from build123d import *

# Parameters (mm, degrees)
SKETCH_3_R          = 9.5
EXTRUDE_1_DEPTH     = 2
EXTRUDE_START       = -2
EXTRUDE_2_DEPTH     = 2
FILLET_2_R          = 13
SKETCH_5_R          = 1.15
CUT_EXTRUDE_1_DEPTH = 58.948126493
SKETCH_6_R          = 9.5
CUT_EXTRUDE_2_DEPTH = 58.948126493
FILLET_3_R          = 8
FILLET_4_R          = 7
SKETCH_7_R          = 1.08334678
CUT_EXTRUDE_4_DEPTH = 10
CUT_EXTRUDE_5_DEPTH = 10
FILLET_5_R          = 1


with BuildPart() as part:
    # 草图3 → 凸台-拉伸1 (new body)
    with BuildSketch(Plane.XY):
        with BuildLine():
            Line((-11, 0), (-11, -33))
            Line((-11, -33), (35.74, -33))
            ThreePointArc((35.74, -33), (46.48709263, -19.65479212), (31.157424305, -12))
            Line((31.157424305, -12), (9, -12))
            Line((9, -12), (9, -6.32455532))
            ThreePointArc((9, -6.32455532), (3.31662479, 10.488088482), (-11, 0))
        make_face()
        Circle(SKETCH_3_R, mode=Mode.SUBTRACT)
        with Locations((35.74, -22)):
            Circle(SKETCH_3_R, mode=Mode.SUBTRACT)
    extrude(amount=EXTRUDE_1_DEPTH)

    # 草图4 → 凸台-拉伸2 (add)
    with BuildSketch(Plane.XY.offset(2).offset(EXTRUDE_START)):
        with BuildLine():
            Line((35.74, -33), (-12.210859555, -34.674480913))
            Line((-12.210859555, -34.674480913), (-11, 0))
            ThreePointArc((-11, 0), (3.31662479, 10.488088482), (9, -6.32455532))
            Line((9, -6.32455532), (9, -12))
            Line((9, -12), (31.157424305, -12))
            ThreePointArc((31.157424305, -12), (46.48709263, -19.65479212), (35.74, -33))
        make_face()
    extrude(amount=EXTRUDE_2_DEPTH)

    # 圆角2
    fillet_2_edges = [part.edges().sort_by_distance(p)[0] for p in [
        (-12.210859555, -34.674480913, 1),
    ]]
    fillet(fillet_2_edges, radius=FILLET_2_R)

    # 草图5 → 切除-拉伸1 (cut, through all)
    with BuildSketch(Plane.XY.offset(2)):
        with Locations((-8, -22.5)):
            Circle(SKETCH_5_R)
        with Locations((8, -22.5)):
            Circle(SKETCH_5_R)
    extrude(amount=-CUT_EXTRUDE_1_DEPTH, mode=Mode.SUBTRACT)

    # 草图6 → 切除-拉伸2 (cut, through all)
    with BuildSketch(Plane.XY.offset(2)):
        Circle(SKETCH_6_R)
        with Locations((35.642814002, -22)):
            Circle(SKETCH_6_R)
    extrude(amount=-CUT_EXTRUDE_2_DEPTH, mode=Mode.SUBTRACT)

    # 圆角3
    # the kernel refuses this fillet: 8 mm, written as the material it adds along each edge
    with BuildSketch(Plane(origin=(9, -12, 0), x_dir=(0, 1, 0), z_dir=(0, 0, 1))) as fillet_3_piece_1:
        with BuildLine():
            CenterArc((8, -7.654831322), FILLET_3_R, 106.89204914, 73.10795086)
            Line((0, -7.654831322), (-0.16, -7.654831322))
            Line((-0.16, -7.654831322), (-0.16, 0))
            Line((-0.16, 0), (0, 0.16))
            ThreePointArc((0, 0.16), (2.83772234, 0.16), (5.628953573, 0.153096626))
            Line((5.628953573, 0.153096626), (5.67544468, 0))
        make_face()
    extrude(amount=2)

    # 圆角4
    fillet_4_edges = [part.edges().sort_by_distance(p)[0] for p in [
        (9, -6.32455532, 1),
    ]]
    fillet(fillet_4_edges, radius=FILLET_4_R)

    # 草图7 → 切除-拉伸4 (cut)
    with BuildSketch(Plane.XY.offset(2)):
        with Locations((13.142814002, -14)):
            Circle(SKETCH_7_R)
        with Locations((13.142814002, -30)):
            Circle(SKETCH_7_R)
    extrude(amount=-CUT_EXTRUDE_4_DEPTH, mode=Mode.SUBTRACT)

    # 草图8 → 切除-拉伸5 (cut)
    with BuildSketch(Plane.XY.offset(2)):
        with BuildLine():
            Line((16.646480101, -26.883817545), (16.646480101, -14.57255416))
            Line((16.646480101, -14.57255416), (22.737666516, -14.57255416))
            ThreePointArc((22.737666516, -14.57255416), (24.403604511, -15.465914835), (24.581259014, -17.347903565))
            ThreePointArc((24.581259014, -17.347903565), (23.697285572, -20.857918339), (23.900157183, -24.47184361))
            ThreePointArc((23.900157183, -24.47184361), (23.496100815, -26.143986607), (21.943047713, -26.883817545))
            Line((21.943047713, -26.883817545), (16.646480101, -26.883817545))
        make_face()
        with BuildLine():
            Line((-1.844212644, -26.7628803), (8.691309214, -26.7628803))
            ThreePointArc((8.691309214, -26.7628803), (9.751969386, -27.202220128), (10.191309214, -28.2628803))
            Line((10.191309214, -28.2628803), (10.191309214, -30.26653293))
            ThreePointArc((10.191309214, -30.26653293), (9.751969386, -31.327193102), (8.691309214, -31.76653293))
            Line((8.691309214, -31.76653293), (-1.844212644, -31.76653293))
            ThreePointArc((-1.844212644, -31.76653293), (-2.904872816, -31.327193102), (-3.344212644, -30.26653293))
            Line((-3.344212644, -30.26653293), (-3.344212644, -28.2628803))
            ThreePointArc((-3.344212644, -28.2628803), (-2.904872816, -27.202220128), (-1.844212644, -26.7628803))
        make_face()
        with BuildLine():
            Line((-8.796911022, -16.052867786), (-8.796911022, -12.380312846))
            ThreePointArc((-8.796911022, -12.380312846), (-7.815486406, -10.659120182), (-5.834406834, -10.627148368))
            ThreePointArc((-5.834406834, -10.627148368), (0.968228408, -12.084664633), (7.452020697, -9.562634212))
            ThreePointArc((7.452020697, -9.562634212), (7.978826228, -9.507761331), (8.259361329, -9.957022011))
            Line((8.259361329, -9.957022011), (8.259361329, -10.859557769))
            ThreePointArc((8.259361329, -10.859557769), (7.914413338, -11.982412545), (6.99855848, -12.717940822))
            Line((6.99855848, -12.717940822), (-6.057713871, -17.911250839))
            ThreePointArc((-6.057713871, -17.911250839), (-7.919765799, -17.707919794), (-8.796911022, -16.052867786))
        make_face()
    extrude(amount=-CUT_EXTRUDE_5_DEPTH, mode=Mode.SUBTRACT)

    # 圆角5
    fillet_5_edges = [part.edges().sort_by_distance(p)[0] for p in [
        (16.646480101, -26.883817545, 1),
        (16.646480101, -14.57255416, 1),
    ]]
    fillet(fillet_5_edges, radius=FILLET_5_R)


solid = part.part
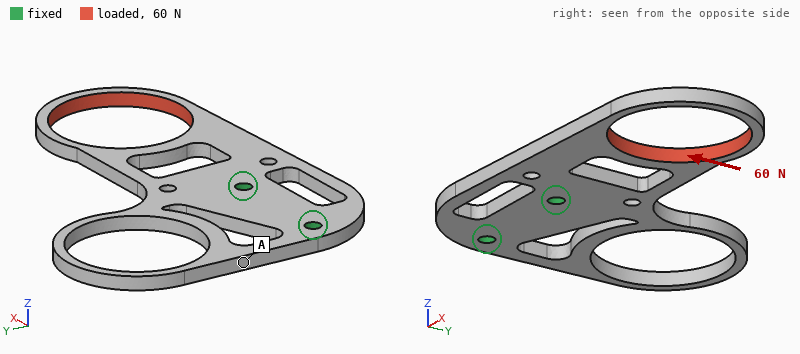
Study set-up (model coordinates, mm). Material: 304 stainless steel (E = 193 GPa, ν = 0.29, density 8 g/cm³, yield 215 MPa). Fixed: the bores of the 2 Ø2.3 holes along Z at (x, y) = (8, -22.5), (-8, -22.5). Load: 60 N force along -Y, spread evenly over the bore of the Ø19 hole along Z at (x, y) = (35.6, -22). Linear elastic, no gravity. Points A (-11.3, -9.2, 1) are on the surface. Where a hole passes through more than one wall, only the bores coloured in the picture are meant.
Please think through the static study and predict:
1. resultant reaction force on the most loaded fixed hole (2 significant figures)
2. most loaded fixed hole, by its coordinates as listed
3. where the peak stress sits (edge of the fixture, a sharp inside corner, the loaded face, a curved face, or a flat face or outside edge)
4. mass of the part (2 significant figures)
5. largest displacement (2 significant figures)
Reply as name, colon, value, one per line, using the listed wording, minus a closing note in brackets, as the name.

resultant reaction force on the most loaded fixed hole: 140 N
most loaded fixed hole, by its coordinates as listed: (8, -22.5)
where the peak stress sits: a curved face
mass of the part: 13 g
largest displacement: 40 µm
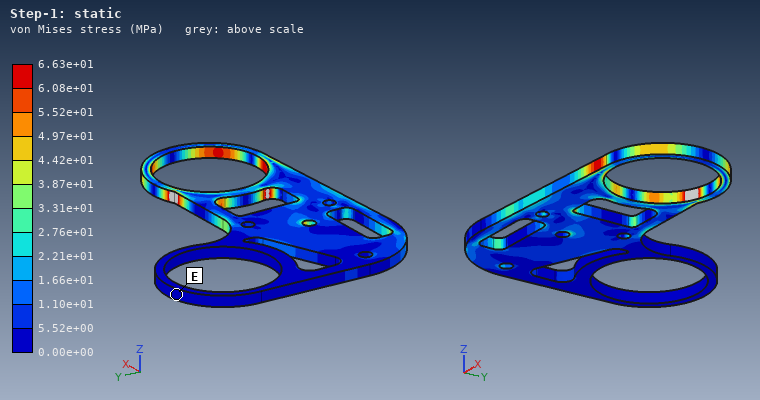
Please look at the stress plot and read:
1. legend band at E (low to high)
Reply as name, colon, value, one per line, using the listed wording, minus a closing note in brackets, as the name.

legend band at E: 0.00e+00 to 5.52e+00 MPa
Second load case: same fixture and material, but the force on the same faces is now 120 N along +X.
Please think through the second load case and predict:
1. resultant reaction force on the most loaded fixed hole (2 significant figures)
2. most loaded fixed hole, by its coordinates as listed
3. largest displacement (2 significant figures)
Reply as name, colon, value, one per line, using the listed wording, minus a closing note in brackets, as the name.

resultant reaction force on the most loaded fixed hole: 90 N
most loaded fixed hole, by its coordinates as listed: (8, -22.5)
largest displacement: 9.5 µm
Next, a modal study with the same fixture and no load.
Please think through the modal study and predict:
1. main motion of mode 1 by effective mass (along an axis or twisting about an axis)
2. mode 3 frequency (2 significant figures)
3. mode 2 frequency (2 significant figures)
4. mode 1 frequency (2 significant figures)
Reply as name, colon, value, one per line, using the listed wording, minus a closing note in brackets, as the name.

main motion of mode 1 by effective mass: along Z
mode 3 frequency: 3400 Hz
mode 2 frequency: 2000 Hz
mode 1 frequency: 1500 Hz
